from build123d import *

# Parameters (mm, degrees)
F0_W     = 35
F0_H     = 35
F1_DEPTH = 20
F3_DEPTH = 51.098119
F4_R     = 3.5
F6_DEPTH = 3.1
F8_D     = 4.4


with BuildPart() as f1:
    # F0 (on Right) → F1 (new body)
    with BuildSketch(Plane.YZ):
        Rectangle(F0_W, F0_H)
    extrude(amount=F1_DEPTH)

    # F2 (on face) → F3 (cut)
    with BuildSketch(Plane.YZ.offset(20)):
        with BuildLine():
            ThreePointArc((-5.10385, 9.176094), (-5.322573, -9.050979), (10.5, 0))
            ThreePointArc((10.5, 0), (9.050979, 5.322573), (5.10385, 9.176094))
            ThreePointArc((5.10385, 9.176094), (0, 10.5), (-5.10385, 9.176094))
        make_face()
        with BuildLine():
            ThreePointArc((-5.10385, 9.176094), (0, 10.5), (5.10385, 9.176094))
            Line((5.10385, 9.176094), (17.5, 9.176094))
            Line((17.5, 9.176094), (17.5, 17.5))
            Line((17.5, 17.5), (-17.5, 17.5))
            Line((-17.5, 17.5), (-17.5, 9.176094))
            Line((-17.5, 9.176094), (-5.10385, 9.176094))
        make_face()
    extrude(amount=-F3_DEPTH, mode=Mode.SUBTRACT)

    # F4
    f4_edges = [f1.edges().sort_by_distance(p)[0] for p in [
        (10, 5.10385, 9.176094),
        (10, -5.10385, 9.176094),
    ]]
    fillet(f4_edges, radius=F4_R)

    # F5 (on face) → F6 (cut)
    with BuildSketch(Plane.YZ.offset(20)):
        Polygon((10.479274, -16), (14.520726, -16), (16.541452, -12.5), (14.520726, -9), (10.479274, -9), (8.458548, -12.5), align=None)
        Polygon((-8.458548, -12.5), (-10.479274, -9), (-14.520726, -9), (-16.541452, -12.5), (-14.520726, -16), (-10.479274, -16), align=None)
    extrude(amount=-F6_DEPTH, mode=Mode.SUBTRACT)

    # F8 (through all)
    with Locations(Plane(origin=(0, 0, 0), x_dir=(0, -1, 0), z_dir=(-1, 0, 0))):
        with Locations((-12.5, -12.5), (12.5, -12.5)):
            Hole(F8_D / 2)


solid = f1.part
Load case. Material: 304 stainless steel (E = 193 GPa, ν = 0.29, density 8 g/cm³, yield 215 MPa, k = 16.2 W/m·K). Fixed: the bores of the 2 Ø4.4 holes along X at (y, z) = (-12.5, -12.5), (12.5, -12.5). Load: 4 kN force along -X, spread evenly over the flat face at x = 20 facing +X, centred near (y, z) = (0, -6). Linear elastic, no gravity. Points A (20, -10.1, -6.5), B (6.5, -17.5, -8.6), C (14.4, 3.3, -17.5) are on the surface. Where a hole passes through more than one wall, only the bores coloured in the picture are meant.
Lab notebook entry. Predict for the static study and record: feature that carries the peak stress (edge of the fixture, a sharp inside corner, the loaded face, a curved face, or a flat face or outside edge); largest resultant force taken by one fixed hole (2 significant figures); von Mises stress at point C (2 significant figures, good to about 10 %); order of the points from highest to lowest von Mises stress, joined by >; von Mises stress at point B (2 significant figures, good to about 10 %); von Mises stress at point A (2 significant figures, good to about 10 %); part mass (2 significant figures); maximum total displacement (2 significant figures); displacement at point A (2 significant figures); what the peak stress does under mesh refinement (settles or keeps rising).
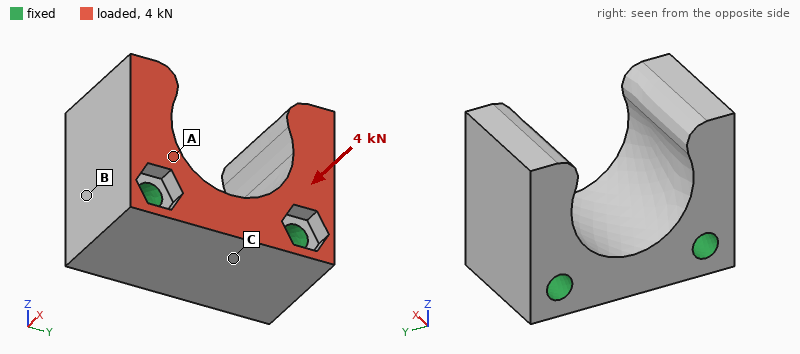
edge of the fixture
2.0 kN
4.9 MPa
A > B > C
10 MPa
17 MPa
86 g
4.0 µm
1.6 µm
keeps rising
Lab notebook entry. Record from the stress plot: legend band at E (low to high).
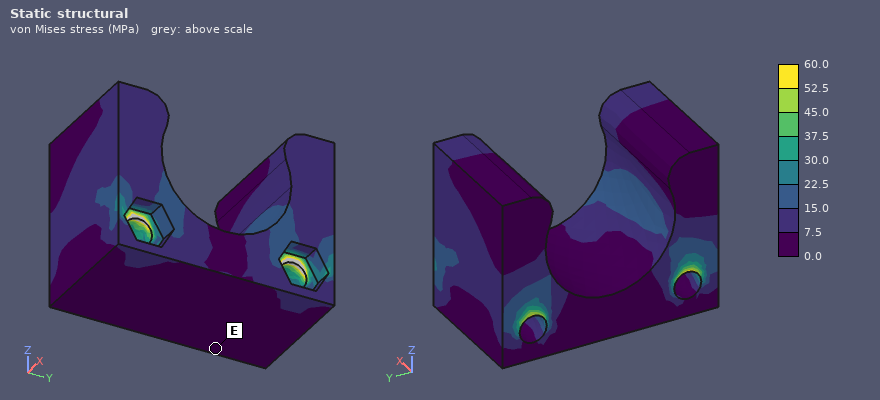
0.0 to 7.5 MPa
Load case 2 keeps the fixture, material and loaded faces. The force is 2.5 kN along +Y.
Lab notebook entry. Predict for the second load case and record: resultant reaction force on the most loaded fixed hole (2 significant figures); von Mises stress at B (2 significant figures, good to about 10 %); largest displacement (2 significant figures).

1.4 kN
19 MPa
9.4 µm
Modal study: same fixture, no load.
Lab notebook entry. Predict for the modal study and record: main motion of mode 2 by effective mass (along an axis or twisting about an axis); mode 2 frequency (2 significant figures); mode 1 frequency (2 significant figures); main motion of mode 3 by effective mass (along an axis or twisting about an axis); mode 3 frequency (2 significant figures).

along Y
15 kHz
14 kHz
along X
23 kHz
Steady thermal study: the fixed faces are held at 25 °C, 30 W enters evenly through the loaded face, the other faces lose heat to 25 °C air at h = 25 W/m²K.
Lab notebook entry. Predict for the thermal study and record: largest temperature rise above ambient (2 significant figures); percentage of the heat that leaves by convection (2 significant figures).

62 K
6.2 %
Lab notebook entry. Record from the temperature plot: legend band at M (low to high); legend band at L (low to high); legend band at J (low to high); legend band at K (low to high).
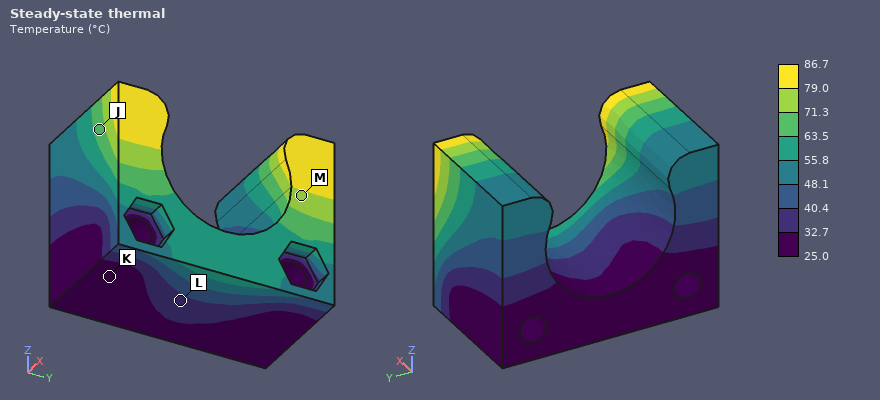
71.3 to 79.0 °C
32.7 to 40.4 °C
63.5 to 71.3 °C
25.0 to 32.7 °C
